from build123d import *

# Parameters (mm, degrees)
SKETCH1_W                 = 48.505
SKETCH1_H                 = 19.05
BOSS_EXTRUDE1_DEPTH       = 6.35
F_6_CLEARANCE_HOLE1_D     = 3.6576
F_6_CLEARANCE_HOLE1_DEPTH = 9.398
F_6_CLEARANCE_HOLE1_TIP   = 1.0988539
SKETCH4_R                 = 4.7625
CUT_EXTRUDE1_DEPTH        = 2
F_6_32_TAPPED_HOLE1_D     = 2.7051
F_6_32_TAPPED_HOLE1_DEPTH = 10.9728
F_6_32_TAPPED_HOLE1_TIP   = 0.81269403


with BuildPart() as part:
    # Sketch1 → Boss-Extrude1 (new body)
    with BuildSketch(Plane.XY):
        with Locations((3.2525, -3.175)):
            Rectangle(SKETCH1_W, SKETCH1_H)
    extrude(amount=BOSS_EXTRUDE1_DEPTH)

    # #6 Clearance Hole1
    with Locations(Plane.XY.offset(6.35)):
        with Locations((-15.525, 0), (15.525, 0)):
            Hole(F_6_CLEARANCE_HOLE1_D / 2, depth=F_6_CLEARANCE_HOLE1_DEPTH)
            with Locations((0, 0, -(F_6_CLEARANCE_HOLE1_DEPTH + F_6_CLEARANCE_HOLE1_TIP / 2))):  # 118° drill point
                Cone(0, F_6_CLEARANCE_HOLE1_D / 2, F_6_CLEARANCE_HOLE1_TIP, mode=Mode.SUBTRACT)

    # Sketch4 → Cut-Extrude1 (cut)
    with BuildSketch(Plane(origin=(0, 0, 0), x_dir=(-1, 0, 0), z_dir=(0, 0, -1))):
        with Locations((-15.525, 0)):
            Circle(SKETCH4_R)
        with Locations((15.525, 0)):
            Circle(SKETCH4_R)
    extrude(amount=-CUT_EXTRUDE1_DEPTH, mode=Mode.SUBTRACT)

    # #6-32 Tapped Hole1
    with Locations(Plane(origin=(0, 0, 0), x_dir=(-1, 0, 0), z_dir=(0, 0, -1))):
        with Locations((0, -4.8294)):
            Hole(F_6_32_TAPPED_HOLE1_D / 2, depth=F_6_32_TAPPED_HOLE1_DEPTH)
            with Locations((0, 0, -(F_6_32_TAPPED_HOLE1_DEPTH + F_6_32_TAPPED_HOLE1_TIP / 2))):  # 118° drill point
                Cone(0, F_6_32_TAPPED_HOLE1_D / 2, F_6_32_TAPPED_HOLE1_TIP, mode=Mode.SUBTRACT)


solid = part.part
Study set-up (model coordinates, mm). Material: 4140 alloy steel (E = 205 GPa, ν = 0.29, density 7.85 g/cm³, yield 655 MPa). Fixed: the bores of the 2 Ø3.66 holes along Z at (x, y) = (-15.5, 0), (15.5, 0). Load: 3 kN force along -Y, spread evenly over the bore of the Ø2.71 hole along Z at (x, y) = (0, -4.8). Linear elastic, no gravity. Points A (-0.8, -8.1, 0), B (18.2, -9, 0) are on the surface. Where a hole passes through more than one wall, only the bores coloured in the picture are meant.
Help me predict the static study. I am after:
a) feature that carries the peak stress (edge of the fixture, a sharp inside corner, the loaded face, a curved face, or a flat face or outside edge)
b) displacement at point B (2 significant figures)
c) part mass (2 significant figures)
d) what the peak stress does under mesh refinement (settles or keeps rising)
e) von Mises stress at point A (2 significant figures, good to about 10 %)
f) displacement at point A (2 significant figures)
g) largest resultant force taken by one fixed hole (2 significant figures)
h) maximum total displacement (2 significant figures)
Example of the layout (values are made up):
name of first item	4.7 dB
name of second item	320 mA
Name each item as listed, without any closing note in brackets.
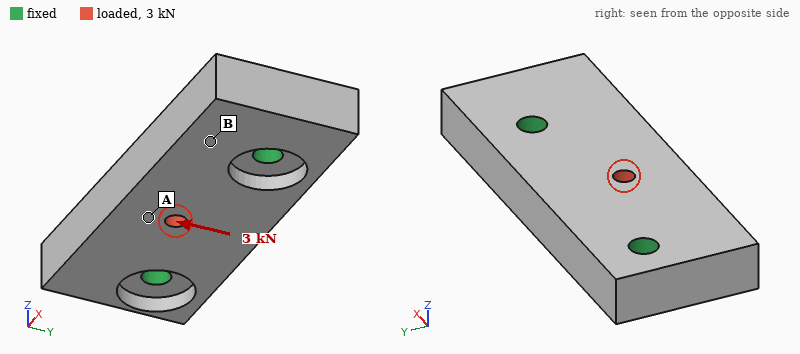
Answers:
feature that carries the peak stress	edge of the fixture
displacement at point B	1.7 µm
part mass	43 g
what the peak stress does under mesh refinement	keeps rising
von Mises stress at point A	42 MPa
displacement at point A	6.0 µm
largest resultant force taken by one fixed hole	1.6 kN
maximum total displacement	6.3 µm
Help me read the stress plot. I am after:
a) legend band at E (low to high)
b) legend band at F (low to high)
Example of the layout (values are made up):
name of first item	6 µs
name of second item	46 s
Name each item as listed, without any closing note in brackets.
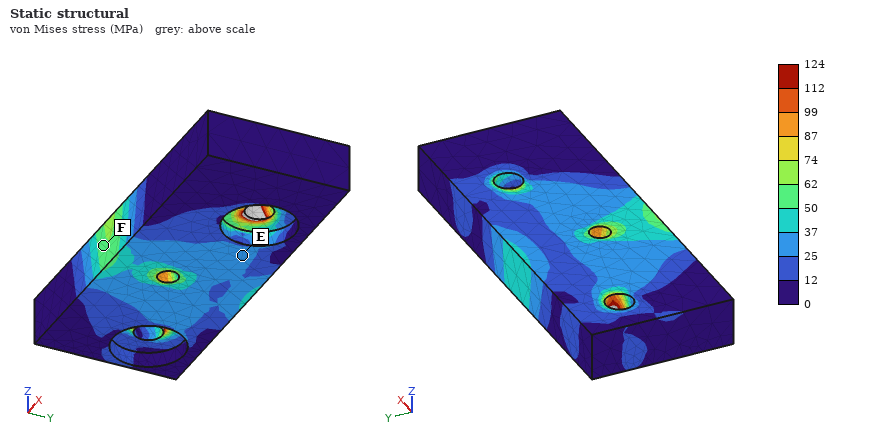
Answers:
legend band at E	25 to 37 MPa
legend band at F	50 to 62 MPa
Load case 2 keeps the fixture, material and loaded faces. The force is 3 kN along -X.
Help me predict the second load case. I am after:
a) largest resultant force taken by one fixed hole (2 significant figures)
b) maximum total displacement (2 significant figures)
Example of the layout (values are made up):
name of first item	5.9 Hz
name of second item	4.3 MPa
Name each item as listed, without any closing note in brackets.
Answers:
largest resultant force taken by one fixed hole	1.6 kN
maximum total displacement	2.7 µm
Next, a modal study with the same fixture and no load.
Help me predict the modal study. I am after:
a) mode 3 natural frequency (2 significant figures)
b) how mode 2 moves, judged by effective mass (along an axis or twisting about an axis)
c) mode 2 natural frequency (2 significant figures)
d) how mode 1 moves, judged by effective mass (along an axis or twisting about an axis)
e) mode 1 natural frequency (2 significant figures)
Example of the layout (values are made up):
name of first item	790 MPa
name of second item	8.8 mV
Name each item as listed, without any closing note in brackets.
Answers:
mode 3 natural frequency	24 kHz
how mode 2 moves, judged by effective mass	twisting about Y
mode 2 natural frequency	18 kHz
how mode 1 moves, judged by effective mass	along Z
mode 1 natural frequency	14 kHz
